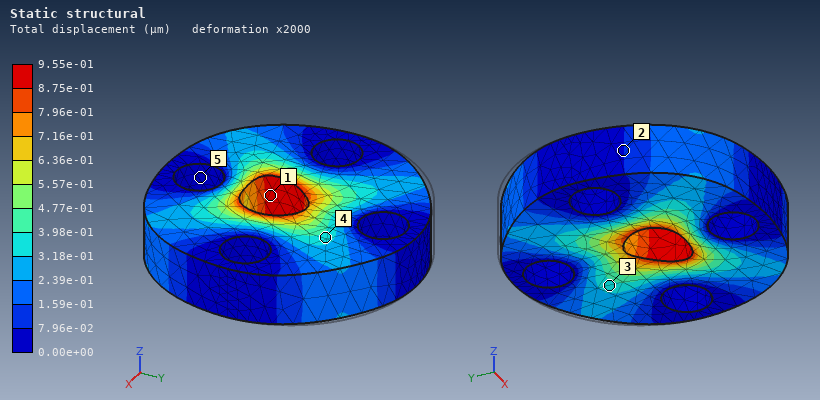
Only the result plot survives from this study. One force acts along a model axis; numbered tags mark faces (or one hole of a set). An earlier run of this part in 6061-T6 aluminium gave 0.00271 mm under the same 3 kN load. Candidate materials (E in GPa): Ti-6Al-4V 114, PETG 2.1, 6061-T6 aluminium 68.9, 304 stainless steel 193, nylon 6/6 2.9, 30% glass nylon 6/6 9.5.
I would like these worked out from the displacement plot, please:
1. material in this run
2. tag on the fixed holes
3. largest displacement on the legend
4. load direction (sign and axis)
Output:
304 stainless steel
5
9.55e-01 µm
-Y
